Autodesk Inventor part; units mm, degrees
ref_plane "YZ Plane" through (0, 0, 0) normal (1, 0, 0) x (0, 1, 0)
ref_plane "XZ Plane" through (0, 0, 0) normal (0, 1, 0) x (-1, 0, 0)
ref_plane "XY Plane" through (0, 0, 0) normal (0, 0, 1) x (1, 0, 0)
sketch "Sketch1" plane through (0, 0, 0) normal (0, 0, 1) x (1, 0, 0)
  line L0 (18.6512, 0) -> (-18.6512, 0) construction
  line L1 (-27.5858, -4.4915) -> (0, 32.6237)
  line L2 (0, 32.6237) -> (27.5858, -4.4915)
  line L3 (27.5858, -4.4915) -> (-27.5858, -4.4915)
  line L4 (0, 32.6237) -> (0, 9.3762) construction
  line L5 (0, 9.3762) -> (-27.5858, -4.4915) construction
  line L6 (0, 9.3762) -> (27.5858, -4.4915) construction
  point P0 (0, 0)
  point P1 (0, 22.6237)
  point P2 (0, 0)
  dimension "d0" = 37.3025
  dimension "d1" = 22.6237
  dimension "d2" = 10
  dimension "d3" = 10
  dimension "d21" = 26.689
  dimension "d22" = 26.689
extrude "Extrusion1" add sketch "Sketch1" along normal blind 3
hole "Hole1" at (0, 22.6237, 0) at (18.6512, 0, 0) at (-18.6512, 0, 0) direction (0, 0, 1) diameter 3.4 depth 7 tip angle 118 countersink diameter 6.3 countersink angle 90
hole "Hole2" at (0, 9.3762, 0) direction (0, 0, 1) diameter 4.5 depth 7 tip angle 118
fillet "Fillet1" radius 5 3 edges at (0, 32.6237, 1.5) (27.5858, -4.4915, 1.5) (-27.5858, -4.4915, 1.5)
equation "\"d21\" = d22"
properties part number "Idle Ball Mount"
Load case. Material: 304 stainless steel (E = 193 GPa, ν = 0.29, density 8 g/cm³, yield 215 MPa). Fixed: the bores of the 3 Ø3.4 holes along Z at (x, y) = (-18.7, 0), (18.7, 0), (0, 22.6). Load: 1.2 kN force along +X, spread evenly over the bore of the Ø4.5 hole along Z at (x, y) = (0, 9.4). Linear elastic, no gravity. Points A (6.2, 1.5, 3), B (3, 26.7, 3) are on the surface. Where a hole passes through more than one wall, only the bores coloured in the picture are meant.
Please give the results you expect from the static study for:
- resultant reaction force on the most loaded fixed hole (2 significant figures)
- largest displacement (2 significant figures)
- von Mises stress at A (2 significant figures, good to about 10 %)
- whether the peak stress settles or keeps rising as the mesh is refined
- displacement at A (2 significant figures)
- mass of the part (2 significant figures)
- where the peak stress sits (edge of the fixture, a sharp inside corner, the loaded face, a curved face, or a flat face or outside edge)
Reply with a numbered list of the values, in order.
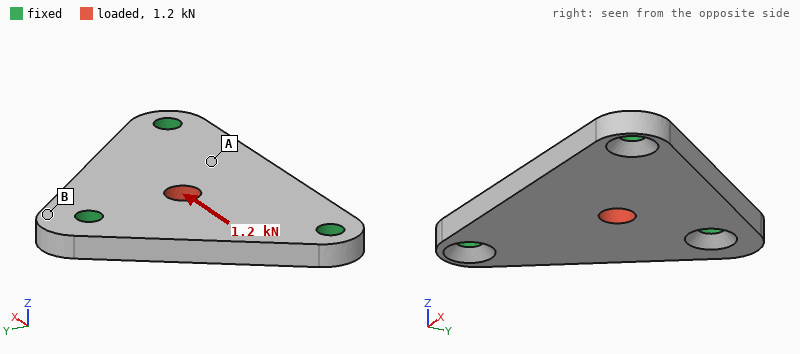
1. 430 N
2. 2.1 µm
3. 12 MPa
4. keeps rising
5. 1.0 µm
6. 22 g
7. edge of the fixture
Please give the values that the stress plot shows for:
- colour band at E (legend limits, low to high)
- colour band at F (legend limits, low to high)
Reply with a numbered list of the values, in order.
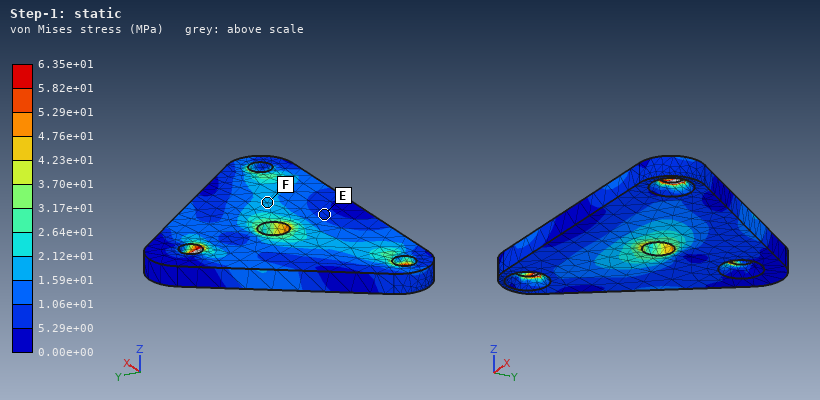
1. 5.29e+00 to 1.06e+01 MPa
2. 1.59e+01 to 2.12e+01 MPa
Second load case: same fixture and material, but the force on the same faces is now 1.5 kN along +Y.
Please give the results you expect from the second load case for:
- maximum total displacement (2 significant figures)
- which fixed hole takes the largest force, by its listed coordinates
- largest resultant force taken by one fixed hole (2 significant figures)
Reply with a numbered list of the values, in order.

1. 3.4 µm
2. (0, 22.6)
3. 950 N
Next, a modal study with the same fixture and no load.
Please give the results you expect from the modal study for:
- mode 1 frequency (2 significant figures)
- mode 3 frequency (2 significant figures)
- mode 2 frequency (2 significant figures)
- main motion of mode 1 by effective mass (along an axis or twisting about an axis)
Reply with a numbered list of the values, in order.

1. 10 kHz
2. 17 kHz
3. 16 kHz
4. along Z
